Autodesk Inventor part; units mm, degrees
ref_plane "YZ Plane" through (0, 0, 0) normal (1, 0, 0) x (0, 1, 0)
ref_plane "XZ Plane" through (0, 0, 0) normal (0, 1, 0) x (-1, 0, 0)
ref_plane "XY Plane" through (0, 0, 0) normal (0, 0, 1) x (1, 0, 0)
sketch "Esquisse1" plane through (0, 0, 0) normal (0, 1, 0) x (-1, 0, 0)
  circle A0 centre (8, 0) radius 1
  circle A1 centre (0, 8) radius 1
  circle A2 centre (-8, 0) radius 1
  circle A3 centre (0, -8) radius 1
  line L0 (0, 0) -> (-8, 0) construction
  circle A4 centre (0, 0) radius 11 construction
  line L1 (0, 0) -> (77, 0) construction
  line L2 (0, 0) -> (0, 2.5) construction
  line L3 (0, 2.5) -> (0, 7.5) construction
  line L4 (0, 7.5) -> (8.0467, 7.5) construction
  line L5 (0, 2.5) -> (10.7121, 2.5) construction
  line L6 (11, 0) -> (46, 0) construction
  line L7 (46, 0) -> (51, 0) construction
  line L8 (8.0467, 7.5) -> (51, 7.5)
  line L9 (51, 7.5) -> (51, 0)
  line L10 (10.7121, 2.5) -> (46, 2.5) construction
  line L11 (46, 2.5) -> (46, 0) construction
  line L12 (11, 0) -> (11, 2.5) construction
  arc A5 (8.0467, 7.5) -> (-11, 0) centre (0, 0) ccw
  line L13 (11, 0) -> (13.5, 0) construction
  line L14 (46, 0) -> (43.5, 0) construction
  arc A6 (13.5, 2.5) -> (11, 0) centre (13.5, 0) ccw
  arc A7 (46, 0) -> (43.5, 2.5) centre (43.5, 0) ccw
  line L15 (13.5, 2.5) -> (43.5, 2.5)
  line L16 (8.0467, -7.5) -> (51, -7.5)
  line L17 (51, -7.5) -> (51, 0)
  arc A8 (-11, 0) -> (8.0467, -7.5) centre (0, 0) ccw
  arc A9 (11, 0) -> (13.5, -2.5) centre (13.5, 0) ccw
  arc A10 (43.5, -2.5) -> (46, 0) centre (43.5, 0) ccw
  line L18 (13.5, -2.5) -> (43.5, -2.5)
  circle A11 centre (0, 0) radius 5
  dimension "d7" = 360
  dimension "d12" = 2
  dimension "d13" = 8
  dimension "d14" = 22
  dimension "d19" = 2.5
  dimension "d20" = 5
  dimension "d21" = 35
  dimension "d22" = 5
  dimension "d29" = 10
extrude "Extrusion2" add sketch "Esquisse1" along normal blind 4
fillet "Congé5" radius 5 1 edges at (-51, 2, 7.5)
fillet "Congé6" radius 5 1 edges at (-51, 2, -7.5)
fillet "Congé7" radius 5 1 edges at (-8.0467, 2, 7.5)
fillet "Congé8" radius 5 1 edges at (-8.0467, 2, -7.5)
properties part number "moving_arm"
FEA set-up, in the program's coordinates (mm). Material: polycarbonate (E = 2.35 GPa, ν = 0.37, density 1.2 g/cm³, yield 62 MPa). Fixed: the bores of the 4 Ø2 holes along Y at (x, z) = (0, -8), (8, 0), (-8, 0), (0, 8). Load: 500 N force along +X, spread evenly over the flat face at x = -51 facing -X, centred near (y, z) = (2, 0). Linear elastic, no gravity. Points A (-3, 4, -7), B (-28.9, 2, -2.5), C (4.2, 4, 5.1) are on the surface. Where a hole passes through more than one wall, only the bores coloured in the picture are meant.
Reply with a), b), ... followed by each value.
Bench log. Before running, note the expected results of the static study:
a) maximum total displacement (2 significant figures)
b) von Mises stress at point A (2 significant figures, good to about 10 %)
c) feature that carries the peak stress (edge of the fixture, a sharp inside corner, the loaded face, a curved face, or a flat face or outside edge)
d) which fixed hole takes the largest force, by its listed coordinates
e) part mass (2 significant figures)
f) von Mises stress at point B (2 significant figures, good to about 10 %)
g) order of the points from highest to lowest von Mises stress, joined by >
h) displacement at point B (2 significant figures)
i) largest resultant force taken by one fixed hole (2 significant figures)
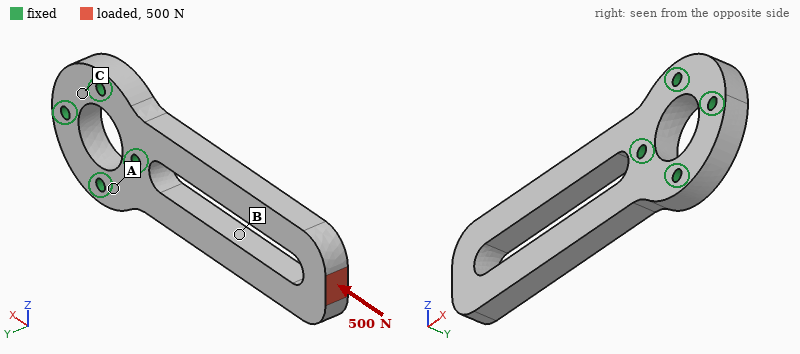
a) 0.35 mm
b) 9.3 MPa
c) a curved face
d) (-8, 0)
e) 3.5 g
f) 18 MPa
g) B > A > C
h) 0.20 mm
i) 200 N
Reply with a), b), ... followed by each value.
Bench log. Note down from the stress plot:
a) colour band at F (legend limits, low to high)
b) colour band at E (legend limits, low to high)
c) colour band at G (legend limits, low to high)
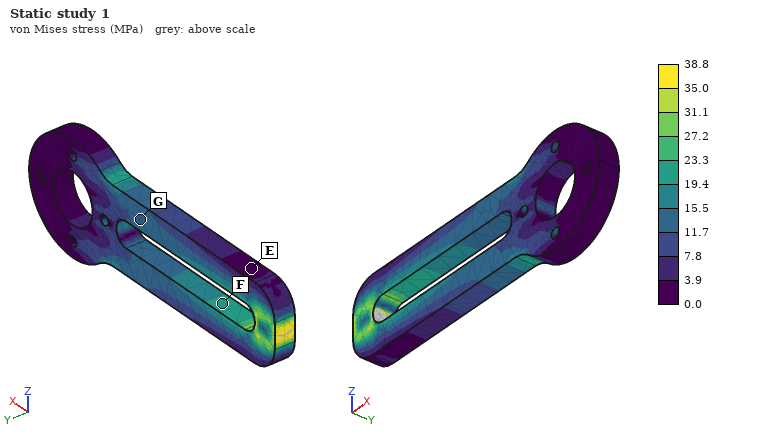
a) 19.4 to 23.3 MPa
b) 0.0 to 3.9 MPa
c) 11.7 to 15.5 MPa
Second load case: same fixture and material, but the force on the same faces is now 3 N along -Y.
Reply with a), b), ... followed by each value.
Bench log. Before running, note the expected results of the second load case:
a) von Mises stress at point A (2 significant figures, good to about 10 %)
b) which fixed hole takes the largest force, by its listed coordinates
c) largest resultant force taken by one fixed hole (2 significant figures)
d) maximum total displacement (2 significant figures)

a) 0.59 MPa
b) (-8, 0)
c) 10 N
d) 0.64 mm
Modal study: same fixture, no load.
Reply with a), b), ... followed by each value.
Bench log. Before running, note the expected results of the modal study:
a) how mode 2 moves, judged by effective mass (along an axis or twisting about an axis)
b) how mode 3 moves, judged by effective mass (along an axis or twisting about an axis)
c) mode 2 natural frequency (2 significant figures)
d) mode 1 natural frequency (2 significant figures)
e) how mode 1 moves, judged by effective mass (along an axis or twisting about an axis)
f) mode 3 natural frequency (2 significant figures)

a) along Z
b) twisting about X
c) 950 Hz
d) 460 Hz
e) along Y
f) 1700 Hz
